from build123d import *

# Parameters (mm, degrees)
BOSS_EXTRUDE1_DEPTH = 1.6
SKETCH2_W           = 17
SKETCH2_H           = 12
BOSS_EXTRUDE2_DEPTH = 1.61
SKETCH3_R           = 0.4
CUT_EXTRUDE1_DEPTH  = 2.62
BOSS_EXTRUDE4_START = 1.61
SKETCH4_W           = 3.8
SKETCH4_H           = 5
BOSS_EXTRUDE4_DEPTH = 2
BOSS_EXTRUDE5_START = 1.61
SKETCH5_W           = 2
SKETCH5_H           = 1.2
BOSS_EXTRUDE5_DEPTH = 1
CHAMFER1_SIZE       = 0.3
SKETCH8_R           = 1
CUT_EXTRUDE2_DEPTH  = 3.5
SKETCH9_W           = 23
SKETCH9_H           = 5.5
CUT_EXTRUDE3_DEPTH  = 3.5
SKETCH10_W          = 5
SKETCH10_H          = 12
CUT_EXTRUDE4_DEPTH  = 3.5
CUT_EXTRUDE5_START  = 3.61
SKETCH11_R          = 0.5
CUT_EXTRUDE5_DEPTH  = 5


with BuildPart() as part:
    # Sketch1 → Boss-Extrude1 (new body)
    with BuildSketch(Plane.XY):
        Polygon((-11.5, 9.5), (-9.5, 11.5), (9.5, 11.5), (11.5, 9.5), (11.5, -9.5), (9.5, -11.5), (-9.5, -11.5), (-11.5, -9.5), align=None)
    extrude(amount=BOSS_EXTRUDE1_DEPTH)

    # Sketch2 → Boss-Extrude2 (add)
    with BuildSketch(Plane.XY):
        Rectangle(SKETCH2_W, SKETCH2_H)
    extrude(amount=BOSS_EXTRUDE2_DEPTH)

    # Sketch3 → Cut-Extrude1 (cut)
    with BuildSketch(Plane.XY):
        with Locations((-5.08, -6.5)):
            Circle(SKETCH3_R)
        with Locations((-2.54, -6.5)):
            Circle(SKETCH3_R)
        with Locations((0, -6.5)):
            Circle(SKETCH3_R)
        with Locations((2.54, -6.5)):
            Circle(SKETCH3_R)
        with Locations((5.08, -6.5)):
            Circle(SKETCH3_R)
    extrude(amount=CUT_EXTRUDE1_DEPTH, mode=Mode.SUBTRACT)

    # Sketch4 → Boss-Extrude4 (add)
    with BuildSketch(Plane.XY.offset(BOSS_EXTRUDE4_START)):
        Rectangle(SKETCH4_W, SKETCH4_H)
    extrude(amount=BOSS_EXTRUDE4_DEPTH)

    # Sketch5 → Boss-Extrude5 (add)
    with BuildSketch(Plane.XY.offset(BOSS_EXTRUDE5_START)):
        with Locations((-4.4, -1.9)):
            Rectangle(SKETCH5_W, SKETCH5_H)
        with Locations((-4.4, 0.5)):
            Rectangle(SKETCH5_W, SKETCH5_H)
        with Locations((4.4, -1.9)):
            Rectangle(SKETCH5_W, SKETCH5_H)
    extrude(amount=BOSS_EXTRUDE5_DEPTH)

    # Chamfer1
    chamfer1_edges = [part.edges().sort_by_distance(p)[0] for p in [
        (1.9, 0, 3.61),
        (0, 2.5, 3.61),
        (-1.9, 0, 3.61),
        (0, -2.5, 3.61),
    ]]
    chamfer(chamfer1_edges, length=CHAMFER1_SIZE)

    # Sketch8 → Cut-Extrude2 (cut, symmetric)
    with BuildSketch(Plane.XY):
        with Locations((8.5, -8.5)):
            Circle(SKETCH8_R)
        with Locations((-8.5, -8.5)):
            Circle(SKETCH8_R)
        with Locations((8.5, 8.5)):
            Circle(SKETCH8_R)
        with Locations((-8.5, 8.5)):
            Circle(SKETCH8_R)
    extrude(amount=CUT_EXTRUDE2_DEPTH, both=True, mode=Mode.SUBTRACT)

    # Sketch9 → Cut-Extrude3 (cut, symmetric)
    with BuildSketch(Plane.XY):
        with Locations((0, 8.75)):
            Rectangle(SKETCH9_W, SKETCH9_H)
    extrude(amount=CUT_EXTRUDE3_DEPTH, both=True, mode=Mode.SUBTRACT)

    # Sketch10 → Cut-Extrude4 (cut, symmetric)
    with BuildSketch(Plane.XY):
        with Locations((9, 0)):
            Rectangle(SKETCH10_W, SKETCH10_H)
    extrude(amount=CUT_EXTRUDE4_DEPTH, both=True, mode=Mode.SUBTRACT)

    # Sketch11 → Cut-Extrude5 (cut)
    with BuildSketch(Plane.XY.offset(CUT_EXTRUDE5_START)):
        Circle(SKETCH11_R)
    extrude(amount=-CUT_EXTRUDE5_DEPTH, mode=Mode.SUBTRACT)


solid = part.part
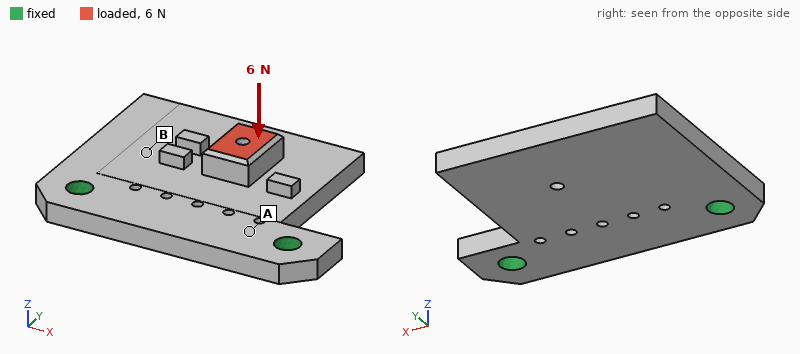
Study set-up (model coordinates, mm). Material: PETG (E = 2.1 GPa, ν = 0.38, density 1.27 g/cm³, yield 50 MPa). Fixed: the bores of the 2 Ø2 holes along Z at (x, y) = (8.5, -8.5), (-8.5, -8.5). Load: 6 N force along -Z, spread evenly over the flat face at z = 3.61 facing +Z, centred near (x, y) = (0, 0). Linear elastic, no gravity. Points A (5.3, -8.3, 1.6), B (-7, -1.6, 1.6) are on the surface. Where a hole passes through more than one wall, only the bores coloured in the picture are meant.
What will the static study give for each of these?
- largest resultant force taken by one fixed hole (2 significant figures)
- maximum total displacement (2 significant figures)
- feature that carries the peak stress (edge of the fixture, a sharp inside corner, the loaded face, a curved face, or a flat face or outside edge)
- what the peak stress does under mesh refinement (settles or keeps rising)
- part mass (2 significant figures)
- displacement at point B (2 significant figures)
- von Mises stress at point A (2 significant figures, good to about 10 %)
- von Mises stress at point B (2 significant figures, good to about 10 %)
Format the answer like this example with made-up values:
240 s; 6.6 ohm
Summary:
3.1 N; 0.32 mm; a sharp inside corner; keeps rising; 0.73 g; 0.090 mm; 5.0 MPa; 2.0 MPa
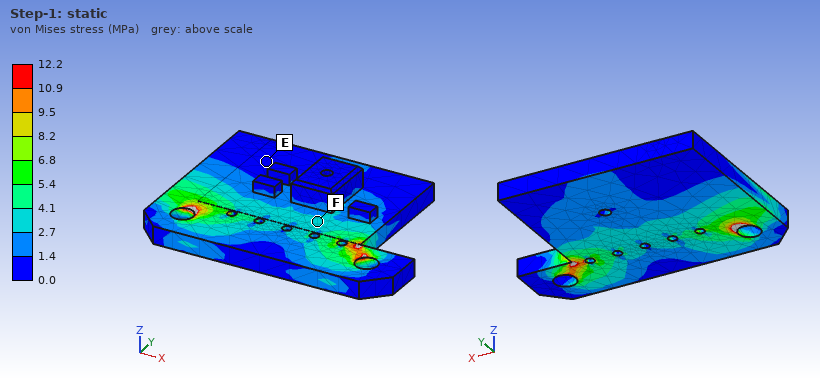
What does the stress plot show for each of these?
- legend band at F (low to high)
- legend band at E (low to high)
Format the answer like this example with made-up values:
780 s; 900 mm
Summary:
2.7 to 4.1 MPa; 0.0 to 1.4 MPa
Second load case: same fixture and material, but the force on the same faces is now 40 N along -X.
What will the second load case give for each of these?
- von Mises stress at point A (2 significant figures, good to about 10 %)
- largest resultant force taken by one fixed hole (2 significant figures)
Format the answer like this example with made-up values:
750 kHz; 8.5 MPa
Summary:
4.5 MPa; 31 N
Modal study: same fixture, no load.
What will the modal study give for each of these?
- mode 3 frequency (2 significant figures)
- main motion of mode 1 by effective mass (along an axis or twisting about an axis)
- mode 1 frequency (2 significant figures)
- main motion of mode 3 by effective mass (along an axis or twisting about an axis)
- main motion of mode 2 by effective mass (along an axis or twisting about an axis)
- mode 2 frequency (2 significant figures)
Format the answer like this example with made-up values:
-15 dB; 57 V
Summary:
7100 Hz; along Z; 1300 Hz; along Z; twisting about Y; 3400 Hz
